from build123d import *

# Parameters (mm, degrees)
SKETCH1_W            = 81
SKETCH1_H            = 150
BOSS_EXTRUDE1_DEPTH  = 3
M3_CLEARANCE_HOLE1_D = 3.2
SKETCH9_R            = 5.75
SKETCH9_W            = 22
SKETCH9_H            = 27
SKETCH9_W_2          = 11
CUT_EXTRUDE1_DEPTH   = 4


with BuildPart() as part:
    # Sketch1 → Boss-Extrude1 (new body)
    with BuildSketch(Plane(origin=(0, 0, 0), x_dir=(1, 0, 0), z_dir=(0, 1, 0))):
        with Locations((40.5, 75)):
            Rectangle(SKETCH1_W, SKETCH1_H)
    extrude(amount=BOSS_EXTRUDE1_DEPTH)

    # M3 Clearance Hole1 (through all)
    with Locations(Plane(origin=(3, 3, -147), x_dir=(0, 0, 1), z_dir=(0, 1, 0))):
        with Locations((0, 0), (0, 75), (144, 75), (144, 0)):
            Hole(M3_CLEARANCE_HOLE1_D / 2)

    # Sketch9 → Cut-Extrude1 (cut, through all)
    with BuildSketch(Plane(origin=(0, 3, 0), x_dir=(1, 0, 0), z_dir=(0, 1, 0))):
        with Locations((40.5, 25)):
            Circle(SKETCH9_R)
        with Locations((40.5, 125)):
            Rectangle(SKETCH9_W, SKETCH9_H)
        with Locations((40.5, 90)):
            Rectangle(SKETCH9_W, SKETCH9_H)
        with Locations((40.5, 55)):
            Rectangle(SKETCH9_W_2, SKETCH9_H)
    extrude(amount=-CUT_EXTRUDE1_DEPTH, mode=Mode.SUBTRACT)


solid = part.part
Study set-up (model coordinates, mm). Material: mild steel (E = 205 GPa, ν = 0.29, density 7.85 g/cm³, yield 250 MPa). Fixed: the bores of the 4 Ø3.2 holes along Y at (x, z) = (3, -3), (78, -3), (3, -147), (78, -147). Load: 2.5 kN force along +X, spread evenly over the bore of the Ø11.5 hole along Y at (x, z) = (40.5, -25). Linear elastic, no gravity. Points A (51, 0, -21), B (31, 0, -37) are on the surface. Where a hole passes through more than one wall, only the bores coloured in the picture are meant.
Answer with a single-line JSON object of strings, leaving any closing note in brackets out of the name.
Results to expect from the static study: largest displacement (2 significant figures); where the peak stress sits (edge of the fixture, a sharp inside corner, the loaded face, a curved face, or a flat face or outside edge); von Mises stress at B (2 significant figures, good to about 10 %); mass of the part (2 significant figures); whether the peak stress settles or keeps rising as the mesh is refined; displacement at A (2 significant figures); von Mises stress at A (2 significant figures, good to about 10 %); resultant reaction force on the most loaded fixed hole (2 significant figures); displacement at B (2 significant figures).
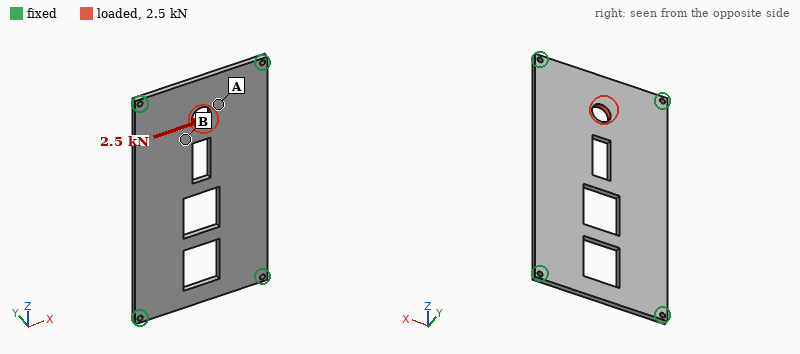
{"largest displacement": "6.8 µm", "where the peak stress sits": "edge of the fixture", "von Mises stress at B": "6.6 MPa", "mass of the part": "250 g", "whether the peak stress settles or keeps rising as the mesh is refined": "keeps rising", "displacement at A": "5.0 µm", "von Mises stress at A": "22 MPa", "resultant reaction force on the most loaded fixed hole": "1.3 kN", "displacement at B": "5.7 µm"}
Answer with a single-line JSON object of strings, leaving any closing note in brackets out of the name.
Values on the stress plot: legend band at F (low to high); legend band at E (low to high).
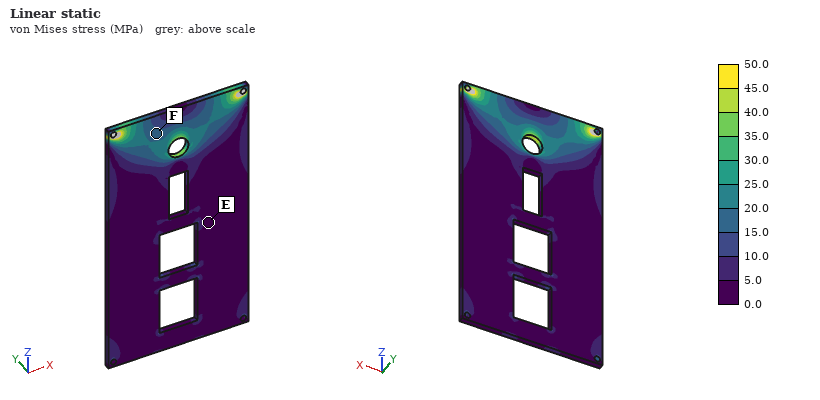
{"legend band at F": "15.0 to 20.0 MPa", "legend band at E": "0.0 to 5.0 MPa"}
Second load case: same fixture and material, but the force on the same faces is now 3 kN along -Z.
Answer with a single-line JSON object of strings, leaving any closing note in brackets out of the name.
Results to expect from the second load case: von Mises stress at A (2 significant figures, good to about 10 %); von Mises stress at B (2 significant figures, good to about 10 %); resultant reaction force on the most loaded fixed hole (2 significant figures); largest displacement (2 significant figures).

{"von Mises stress at A": "19 MPa", "von Mises stress at B": "27 MPa", "resultant reaction force on the most loaded fixed hole": "1.2 kN", "largest displacement": "8.1 µm"}
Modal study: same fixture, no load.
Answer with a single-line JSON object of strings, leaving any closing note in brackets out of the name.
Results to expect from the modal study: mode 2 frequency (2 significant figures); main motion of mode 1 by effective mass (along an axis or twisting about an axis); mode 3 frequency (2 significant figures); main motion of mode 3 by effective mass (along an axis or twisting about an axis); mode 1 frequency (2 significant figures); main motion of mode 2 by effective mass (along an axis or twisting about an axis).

{"mode 2 frequency": "1100 Hz", "main motion of mode 1 by effective mass": "along Y", "mode 3 frequency": "1600 Hz", "main motion of mode 3 by effective mass": "twisting about X", "mode 1 frequency": "590 Hz", "main motion of mode 2 by effective mass": "twisting about Z"}
